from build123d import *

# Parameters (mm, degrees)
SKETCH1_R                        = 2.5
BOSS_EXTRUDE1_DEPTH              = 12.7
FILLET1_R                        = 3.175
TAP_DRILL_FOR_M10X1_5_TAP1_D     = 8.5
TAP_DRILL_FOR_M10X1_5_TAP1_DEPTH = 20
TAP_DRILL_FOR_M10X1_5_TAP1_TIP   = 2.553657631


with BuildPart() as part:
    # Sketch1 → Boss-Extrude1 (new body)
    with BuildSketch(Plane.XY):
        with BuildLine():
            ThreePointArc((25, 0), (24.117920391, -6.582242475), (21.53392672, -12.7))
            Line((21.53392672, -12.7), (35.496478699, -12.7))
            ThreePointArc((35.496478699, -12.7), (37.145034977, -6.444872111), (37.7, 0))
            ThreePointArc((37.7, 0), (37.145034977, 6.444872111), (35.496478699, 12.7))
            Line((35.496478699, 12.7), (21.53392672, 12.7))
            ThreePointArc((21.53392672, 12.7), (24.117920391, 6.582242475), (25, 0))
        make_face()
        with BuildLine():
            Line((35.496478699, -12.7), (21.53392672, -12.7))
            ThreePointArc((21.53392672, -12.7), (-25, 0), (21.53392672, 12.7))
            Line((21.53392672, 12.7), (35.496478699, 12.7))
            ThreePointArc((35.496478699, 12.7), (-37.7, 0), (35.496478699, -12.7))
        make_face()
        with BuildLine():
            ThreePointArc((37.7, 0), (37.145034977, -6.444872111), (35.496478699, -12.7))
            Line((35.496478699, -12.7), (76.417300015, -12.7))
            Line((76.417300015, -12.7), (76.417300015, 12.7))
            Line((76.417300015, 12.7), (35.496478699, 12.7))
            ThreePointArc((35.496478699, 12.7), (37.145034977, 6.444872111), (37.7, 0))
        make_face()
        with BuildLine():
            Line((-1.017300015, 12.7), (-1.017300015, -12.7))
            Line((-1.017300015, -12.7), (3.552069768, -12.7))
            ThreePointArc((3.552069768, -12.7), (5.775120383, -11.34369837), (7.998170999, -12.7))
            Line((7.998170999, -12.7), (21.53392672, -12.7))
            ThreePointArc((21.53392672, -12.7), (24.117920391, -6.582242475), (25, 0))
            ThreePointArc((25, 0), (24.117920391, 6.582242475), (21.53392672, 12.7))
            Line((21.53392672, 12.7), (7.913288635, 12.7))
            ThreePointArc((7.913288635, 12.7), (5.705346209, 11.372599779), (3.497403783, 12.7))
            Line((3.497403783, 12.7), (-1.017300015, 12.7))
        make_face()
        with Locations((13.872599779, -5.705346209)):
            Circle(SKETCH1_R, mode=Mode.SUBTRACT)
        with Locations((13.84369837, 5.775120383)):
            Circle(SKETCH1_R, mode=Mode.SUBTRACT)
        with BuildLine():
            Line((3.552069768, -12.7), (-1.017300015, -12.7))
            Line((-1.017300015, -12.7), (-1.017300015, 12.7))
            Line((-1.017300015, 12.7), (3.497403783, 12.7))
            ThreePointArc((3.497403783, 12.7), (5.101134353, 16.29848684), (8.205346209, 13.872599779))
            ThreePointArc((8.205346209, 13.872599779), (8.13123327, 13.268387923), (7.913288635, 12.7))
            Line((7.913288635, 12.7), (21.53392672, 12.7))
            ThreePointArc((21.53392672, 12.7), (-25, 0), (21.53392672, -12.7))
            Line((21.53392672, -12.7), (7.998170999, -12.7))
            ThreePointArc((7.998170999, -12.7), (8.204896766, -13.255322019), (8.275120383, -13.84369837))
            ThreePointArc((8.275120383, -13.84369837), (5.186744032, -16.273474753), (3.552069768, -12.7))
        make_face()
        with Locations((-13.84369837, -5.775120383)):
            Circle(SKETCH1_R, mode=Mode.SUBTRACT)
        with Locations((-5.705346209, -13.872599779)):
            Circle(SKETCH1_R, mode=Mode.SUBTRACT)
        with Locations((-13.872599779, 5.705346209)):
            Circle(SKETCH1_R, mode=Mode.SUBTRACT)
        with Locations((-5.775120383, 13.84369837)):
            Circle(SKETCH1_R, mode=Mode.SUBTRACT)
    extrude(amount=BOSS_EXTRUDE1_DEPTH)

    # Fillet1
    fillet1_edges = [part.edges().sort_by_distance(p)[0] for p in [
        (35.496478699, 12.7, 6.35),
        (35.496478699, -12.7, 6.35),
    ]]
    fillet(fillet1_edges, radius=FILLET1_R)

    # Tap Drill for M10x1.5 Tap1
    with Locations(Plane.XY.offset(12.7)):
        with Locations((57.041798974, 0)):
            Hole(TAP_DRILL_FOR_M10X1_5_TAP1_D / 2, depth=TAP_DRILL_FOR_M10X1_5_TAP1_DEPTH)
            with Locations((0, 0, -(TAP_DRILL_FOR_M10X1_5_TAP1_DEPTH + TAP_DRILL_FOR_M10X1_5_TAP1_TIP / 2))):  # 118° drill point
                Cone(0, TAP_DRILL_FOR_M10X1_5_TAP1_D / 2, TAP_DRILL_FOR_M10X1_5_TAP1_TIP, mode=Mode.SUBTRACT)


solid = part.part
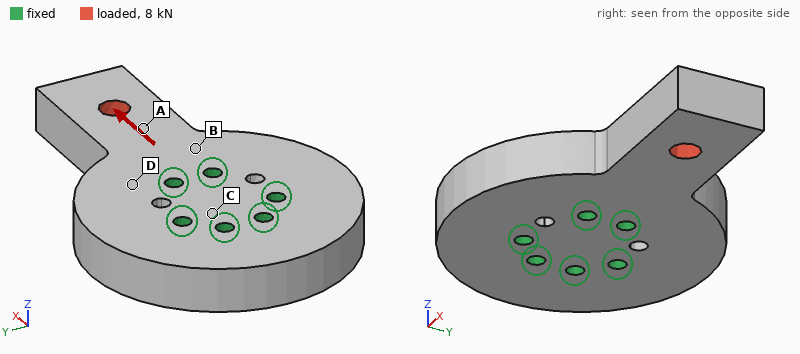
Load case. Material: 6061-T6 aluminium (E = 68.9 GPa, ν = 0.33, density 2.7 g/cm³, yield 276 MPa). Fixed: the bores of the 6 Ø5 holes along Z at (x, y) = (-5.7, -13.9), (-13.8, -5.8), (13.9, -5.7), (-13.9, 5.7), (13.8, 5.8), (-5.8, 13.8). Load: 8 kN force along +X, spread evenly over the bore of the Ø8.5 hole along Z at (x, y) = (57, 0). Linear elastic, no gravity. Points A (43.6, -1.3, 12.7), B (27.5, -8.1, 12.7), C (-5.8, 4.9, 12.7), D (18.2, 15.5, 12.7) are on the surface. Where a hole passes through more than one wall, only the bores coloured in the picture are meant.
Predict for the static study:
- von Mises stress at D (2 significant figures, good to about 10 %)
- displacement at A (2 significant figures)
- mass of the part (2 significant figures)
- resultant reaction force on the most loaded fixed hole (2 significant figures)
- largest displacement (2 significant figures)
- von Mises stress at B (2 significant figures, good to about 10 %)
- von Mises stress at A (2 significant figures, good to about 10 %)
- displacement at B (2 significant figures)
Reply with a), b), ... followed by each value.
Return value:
a) 7.5 MPa
b) 9.1 µm
c) 180 g
d) 3.3 kN
e) 18 µm
f) 21 MPa
g) 24 MPa
h) 4.0 µm
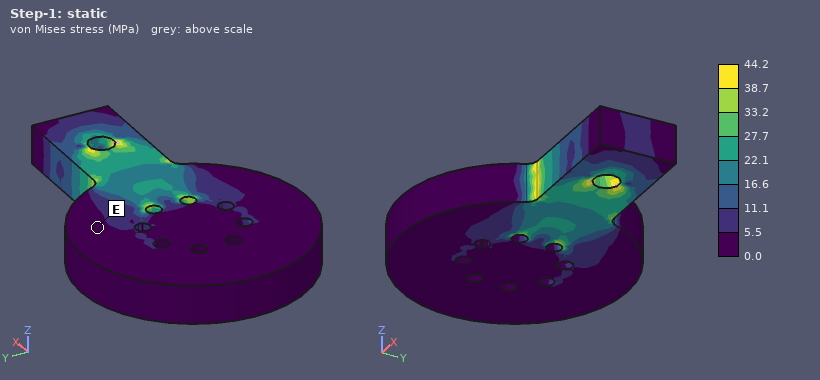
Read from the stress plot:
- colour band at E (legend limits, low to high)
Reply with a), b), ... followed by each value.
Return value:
a) 0.0 to 5.5 MPa
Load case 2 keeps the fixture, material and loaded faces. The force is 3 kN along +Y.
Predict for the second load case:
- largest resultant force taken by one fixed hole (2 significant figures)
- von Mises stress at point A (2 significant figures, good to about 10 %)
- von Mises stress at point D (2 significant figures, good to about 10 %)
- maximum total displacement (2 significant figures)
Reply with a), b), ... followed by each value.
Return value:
a) 3.2 kN
b) 25 MPa
c) 15 MPa
d) 70 µm
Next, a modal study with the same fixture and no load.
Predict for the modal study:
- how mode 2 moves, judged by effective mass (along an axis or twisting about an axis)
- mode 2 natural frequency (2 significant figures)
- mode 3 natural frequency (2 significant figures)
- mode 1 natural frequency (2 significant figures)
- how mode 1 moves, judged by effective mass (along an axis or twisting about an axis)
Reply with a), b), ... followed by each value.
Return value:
a) along Y
b) 6600 Hz
c) 10 kHz
d) 3100 Hz
e) along Z
